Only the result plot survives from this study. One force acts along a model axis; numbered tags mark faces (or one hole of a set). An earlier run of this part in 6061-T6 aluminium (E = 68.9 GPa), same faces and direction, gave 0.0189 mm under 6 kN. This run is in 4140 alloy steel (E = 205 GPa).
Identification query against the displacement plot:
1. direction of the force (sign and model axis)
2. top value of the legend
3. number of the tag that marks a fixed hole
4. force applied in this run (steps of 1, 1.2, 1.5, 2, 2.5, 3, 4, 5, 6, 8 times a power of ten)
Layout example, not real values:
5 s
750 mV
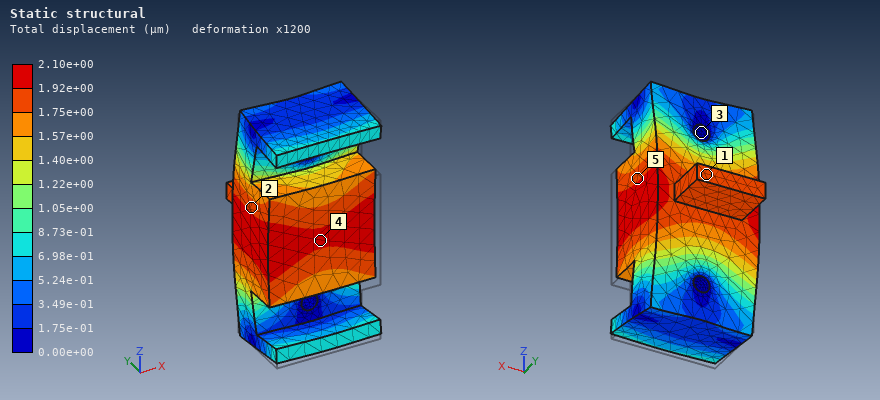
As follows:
+Y
2.10e+00 µm
3
2 kN
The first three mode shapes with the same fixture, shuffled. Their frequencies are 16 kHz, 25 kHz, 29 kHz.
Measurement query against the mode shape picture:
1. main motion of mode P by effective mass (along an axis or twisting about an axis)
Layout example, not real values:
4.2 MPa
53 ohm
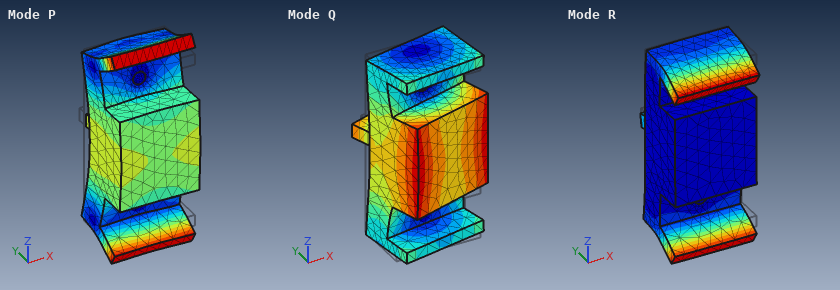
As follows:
along Y
